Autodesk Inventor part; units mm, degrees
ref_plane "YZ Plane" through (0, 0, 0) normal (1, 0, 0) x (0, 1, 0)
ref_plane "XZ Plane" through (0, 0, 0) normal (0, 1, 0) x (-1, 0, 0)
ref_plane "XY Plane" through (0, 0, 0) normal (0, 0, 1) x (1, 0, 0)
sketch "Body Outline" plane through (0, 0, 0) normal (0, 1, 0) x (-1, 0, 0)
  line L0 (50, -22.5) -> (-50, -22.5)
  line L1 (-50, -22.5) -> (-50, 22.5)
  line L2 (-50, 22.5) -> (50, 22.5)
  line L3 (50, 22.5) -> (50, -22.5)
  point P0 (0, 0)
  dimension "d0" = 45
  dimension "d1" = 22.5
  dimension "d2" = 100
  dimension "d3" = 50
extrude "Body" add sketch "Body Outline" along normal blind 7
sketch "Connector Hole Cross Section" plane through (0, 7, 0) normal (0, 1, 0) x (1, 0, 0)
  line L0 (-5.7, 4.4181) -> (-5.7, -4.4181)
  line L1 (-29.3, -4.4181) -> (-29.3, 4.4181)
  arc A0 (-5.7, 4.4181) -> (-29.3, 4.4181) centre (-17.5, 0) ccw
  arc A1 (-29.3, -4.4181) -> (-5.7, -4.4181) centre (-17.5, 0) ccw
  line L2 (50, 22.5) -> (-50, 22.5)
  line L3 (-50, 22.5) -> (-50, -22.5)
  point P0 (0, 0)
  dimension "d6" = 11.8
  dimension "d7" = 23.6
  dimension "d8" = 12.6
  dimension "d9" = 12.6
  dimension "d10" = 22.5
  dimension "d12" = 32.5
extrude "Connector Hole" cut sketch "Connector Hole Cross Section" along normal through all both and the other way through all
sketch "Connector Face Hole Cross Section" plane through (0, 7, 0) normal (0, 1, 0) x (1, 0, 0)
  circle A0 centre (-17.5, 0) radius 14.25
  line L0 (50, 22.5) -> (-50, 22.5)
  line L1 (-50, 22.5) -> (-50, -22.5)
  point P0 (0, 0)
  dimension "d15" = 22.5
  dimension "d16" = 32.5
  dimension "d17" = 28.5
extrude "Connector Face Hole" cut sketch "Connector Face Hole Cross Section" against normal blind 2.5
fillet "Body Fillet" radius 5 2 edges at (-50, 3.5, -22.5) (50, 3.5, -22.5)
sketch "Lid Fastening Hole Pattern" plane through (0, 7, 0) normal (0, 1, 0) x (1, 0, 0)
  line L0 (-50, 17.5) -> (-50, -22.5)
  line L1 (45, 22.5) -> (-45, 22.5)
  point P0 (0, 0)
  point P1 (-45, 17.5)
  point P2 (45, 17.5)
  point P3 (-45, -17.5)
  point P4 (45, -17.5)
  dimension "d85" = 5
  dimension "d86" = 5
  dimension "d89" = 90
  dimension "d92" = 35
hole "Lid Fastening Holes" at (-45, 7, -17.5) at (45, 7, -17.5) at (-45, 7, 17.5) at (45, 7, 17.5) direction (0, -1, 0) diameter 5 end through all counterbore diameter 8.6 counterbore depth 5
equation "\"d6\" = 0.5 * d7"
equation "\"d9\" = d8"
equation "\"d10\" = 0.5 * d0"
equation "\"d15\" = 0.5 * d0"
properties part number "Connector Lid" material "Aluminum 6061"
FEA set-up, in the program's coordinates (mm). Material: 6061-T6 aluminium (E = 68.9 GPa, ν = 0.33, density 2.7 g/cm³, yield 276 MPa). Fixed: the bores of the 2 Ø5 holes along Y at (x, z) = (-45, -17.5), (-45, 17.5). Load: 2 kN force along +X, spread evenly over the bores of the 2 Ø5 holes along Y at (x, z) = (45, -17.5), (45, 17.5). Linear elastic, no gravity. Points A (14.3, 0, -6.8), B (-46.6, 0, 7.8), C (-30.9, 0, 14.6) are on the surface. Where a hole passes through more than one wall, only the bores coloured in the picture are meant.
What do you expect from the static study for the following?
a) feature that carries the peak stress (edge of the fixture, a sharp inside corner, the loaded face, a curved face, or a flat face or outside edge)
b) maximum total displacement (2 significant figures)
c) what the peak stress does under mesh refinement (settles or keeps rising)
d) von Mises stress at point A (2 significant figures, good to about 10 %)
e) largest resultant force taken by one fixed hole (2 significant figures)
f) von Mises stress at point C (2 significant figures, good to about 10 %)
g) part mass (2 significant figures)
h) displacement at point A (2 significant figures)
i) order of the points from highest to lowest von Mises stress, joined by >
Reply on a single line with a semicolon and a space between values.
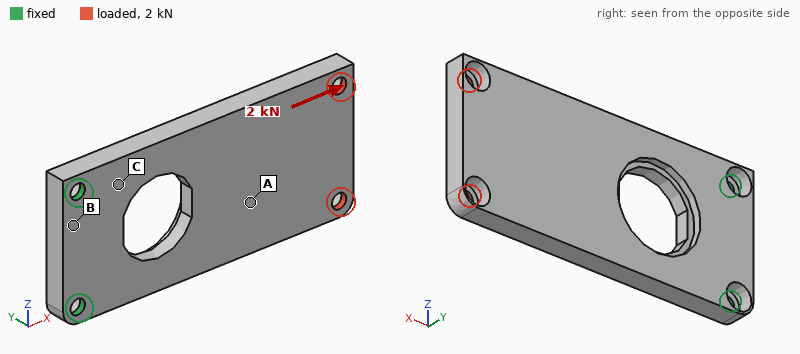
a sharp inside corner; 0.36 mm; keeps rising; 17 MPa; 1.0 kN; 33 MPa; 71 g; 0.15 mm; C > A > B
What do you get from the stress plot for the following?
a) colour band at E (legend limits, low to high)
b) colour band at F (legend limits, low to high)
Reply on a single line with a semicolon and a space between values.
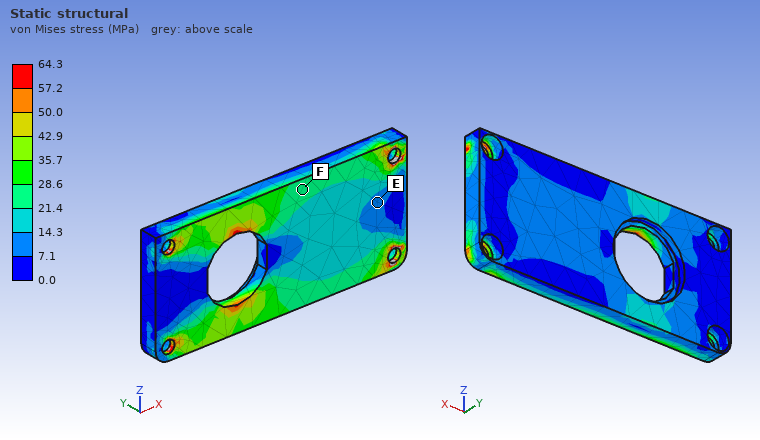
7.1 to 14.3 MPa; 21.4 to 28.6 MPa
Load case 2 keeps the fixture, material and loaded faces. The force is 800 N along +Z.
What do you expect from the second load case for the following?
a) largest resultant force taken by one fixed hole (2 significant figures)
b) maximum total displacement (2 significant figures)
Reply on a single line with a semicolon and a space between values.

2.0 kN; 0.16 mm
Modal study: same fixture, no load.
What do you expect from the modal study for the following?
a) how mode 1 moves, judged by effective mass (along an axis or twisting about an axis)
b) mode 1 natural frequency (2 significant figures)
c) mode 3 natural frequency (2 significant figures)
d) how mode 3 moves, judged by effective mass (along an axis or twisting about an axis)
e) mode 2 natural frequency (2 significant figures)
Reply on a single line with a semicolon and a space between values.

along Y; 380 Hz; 2600 Hz; along Z; 2100 Hz
